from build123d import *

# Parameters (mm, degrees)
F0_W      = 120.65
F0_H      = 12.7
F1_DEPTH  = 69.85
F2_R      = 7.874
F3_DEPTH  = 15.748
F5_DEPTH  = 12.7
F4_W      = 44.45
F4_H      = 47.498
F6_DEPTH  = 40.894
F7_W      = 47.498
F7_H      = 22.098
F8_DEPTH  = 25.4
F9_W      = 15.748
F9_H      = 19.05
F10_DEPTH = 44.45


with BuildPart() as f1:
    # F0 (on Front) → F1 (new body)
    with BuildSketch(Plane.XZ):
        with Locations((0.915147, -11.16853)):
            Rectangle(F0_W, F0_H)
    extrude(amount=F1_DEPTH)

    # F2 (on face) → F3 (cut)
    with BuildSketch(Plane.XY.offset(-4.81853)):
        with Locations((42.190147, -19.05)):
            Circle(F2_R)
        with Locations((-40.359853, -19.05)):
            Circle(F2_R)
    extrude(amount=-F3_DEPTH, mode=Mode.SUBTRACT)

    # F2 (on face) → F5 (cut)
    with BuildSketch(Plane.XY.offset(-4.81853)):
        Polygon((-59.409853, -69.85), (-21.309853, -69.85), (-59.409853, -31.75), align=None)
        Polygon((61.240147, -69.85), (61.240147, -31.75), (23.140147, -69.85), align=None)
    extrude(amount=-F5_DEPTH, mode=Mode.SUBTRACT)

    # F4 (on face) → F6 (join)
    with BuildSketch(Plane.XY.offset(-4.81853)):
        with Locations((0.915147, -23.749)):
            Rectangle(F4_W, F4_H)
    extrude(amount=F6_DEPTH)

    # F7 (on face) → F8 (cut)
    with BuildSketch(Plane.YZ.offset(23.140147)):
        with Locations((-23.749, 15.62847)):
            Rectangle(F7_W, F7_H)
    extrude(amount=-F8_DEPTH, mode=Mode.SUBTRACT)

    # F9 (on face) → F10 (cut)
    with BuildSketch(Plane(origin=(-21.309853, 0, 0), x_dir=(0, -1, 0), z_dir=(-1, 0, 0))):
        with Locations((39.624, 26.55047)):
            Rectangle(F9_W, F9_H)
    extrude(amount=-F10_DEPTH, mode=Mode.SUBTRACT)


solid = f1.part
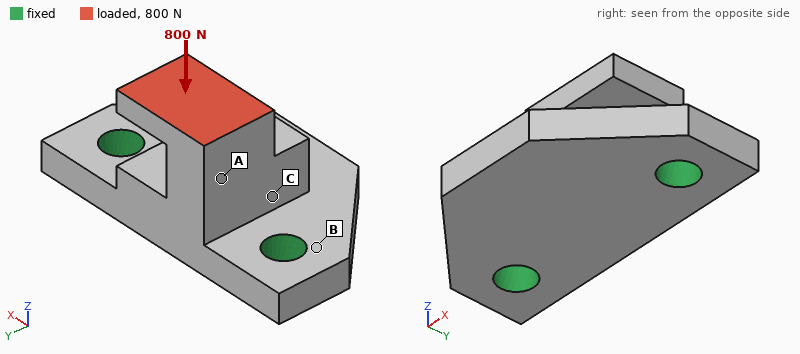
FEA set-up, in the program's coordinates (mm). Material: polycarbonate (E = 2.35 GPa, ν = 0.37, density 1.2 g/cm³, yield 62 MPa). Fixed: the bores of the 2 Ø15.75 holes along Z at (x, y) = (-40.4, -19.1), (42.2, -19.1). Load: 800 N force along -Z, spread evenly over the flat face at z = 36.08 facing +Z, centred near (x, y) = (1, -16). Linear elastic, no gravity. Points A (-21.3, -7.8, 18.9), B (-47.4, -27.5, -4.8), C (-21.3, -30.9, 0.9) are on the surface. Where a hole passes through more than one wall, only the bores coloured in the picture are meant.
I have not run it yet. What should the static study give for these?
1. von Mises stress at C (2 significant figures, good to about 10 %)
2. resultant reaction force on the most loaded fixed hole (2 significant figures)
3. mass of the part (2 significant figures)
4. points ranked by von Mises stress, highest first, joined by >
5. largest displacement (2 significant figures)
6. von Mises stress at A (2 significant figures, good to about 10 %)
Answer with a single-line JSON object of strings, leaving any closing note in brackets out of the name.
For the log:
{"von Mises stress at C": "1.7 MPa", "resultant reaction force on the most loaded fixed hole": "470 N", "mass of the part": "160 g", "points ranked by von Mises stress, highest first, joined by >": "A > C > B", "largest displacement": "0.74 mm", "von Mises stress at A": "3.4 MPa"}
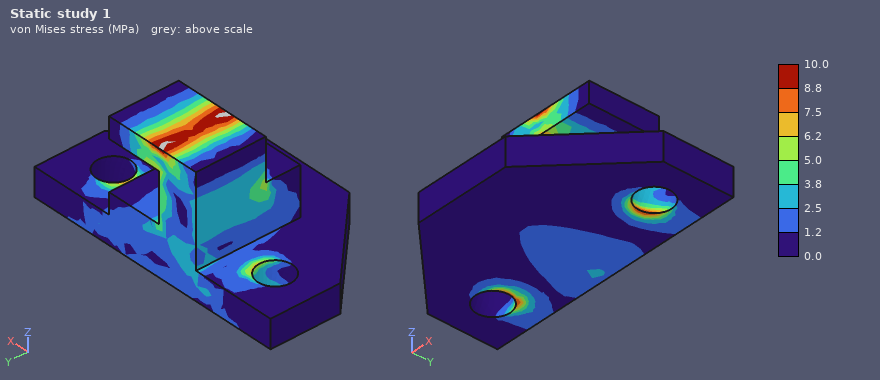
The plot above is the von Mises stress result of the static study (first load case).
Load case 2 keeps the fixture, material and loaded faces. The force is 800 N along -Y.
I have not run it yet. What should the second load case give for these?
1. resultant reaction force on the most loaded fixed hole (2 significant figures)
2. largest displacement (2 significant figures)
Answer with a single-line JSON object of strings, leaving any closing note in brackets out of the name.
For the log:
{"resultant reaction force on the most loaded fixed hole": "450 N", "largest displacement": "0.98 mm"}
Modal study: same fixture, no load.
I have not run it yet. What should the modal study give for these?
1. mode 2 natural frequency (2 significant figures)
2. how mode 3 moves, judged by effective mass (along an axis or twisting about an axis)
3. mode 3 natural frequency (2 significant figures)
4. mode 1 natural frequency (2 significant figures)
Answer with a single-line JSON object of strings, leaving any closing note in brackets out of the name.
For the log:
{"mode 2 natural frequency": "1300 Hz", "how mode 3 moves, judged by effective mass": "along Z", "mode 3 natural frequency": "1900 Hz", "mode 1 natural frequency": "930 Hz"}
